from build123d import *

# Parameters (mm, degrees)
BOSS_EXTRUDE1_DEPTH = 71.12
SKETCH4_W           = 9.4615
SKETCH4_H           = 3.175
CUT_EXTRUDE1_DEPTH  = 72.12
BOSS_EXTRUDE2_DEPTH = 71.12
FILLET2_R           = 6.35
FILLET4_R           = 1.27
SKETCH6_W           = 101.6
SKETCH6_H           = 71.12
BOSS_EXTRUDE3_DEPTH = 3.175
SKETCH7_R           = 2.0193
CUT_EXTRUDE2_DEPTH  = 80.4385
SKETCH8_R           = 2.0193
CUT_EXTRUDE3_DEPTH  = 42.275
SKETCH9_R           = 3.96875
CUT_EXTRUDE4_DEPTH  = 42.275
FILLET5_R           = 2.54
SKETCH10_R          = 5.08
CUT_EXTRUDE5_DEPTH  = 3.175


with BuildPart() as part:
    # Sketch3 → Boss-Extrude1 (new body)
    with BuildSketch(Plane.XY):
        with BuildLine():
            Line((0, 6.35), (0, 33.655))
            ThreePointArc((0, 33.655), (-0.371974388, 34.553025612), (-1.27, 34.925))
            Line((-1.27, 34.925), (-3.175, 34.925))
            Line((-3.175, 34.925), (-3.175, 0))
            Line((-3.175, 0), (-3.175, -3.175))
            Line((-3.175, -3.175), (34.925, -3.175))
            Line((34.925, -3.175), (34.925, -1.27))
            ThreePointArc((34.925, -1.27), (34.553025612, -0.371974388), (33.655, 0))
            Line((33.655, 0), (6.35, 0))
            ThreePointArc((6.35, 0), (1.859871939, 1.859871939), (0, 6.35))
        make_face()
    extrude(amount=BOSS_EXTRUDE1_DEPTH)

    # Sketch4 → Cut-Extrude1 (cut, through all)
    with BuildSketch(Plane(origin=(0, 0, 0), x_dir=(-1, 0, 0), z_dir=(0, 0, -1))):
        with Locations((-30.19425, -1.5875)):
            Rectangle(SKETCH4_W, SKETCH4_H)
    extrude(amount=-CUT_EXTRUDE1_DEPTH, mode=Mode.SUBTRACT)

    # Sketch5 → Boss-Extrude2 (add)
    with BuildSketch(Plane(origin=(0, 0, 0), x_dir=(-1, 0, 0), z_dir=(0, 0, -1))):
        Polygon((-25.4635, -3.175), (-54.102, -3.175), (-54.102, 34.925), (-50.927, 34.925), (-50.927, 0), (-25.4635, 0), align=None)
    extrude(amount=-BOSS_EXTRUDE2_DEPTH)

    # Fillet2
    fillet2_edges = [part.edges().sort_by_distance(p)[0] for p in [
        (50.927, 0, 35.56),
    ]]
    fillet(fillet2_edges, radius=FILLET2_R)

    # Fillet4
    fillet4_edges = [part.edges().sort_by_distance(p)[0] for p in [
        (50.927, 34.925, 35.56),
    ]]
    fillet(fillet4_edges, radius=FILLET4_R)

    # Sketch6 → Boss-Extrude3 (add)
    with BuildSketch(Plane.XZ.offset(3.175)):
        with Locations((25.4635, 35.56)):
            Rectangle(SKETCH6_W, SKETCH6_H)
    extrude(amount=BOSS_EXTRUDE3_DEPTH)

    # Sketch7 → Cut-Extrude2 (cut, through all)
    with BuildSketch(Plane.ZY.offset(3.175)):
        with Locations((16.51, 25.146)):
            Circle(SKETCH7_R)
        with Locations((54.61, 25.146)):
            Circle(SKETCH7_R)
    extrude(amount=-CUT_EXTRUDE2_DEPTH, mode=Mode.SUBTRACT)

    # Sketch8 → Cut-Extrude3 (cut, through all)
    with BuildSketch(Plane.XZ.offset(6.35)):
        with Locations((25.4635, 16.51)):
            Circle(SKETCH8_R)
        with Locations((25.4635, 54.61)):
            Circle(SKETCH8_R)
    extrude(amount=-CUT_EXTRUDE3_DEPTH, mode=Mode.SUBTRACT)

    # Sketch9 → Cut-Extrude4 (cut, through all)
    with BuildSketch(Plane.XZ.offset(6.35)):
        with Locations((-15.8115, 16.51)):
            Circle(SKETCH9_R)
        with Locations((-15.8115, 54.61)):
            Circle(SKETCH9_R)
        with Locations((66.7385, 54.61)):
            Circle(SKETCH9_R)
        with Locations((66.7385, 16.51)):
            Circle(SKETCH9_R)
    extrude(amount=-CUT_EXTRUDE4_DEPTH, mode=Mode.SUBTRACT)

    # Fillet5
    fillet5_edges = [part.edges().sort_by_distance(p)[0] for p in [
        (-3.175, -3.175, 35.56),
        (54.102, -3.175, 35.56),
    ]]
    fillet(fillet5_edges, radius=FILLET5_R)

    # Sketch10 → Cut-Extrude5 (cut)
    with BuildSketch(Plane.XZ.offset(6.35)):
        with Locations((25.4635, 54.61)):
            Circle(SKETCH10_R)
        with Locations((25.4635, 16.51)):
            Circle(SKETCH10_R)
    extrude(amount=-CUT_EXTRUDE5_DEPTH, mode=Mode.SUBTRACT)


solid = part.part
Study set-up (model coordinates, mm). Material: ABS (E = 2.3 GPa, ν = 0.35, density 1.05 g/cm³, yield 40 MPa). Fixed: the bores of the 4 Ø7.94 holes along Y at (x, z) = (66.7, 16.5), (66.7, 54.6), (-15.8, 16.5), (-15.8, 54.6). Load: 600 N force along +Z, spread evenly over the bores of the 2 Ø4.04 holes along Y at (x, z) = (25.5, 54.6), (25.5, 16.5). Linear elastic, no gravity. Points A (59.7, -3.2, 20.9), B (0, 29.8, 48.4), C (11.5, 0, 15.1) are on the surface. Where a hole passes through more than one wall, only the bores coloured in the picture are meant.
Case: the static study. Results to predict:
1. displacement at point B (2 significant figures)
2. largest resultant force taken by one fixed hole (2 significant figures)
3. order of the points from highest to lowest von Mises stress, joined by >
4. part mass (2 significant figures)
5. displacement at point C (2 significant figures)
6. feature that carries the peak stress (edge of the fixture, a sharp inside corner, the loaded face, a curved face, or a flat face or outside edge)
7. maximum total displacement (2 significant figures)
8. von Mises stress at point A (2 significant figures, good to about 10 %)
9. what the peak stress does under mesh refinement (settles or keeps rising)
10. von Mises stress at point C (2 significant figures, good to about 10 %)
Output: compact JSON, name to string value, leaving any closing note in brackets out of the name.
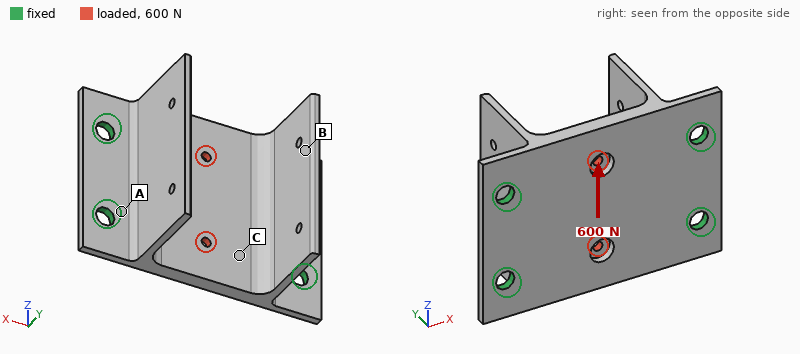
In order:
{"displacement at point B": "0.081 mm", "largest resultant force taken by one fixed hole": "170 N", "order of the points from highest to lowest von Mises stress, joined by >": "A > C > B", "part mass": "54 g", "displacement at point C": "0.067 mm", "feature that carries the peak stress": "a sharp inside corner", "maximum total displacement": "0.12 mm", "von Mises stress at point A": "4.3 MPa", "what the peak stress does under mesh refinement": "keeps rising", "von Mises stress at point C": "1.6 MPa"}
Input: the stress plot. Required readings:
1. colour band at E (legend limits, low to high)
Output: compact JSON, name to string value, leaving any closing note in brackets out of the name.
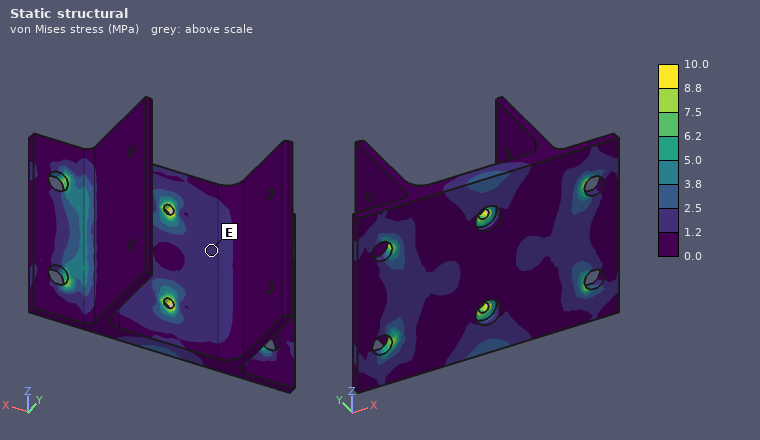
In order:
{"colour band at E": "1.2 to 2.5 MPa"}
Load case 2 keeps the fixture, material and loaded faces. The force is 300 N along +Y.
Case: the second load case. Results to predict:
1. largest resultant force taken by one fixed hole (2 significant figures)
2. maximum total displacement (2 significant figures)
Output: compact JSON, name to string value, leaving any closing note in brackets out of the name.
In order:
{"largest resultant force taken by one fixed hole": "210 N", "maximum total displacement": "0.60 mm"}
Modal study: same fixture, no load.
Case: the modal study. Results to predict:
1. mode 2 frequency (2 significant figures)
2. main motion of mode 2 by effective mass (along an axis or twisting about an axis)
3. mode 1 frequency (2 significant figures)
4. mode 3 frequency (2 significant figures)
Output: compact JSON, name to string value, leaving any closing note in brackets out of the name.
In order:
{"mode 2 frequency": "710 Hz", "main motion of mode 2 by effective mass": "along X", "mode 1 frequency": "600 Hz", "mode 3 frequency": "870 Hz"}
